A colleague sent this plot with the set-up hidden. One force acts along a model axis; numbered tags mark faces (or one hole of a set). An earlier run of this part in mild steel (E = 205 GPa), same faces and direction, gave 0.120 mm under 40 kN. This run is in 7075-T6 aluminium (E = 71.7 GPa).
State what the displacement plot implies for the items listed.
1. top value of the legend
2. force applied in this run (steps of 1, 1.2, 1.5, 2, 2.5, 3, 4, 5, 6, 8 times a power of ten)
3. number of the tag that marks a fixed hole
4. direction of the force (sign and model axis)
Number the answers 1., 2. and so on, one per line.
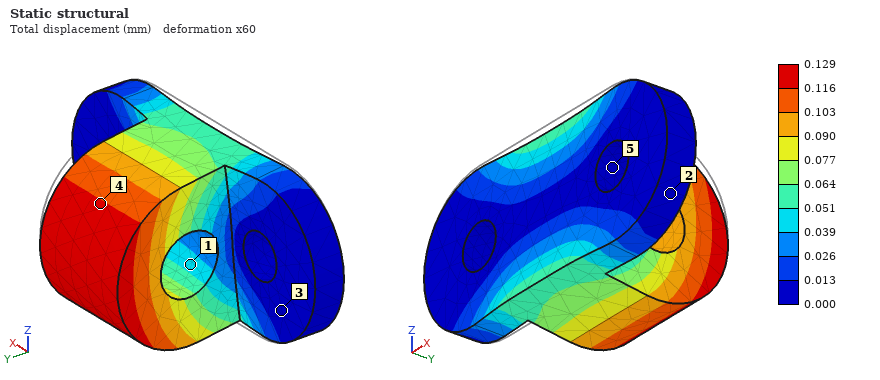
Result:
1. 0.129 mm
2. 15 kN
3. 5
4. -Z
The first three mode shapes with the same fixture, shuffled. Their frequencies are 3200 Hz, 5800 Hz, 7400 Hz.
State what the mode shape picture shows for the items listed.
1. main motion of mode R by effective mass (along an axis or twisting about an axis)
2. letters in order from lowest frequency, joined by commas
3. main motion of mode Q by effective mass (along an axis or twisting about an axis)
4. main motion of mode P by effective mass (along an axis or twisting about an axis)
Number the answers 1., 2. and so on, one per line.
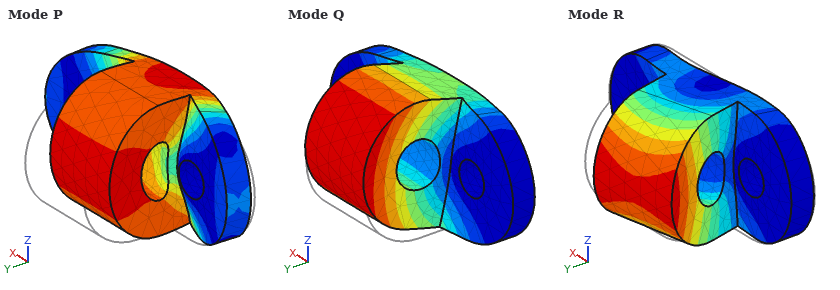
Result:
1. along X
2. Q, R, P
3. along Z
4. along Y
